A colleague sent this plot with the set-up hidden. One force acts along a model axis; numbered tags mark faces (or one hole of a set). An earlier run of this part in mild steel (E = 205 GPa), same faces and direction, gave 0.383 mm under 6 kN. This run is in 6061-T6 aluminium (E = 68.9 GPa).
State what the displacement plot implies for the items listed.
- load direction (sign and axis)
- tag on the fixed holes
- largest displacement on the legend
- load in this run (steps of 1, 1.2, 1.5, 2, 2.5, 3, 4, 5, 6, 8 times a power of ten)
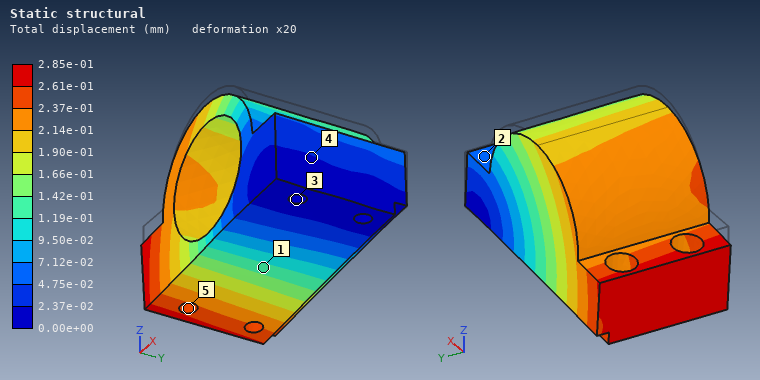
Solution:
-Z
3
2.85e-01 mm
1.5 kN
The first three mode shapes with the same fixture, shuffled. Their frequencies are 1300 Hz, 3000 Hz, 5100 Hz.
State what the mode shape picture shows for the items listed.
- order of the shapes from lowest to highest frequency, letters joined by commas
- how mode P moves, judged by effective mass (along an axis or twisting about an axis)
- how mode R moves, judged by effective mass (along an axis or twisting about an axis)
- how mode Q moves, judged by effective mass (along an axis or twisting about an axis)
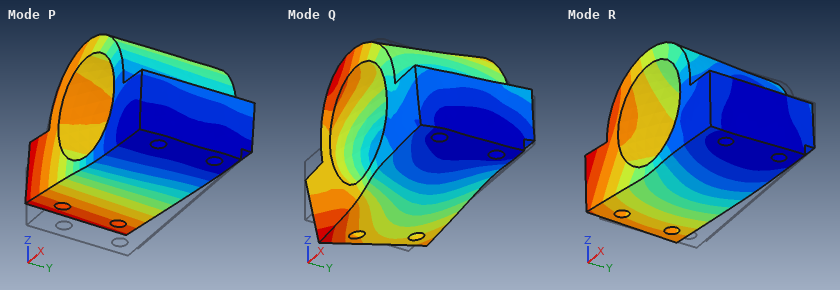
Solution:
P, R, Q
along Z
along Y
twisting about X
